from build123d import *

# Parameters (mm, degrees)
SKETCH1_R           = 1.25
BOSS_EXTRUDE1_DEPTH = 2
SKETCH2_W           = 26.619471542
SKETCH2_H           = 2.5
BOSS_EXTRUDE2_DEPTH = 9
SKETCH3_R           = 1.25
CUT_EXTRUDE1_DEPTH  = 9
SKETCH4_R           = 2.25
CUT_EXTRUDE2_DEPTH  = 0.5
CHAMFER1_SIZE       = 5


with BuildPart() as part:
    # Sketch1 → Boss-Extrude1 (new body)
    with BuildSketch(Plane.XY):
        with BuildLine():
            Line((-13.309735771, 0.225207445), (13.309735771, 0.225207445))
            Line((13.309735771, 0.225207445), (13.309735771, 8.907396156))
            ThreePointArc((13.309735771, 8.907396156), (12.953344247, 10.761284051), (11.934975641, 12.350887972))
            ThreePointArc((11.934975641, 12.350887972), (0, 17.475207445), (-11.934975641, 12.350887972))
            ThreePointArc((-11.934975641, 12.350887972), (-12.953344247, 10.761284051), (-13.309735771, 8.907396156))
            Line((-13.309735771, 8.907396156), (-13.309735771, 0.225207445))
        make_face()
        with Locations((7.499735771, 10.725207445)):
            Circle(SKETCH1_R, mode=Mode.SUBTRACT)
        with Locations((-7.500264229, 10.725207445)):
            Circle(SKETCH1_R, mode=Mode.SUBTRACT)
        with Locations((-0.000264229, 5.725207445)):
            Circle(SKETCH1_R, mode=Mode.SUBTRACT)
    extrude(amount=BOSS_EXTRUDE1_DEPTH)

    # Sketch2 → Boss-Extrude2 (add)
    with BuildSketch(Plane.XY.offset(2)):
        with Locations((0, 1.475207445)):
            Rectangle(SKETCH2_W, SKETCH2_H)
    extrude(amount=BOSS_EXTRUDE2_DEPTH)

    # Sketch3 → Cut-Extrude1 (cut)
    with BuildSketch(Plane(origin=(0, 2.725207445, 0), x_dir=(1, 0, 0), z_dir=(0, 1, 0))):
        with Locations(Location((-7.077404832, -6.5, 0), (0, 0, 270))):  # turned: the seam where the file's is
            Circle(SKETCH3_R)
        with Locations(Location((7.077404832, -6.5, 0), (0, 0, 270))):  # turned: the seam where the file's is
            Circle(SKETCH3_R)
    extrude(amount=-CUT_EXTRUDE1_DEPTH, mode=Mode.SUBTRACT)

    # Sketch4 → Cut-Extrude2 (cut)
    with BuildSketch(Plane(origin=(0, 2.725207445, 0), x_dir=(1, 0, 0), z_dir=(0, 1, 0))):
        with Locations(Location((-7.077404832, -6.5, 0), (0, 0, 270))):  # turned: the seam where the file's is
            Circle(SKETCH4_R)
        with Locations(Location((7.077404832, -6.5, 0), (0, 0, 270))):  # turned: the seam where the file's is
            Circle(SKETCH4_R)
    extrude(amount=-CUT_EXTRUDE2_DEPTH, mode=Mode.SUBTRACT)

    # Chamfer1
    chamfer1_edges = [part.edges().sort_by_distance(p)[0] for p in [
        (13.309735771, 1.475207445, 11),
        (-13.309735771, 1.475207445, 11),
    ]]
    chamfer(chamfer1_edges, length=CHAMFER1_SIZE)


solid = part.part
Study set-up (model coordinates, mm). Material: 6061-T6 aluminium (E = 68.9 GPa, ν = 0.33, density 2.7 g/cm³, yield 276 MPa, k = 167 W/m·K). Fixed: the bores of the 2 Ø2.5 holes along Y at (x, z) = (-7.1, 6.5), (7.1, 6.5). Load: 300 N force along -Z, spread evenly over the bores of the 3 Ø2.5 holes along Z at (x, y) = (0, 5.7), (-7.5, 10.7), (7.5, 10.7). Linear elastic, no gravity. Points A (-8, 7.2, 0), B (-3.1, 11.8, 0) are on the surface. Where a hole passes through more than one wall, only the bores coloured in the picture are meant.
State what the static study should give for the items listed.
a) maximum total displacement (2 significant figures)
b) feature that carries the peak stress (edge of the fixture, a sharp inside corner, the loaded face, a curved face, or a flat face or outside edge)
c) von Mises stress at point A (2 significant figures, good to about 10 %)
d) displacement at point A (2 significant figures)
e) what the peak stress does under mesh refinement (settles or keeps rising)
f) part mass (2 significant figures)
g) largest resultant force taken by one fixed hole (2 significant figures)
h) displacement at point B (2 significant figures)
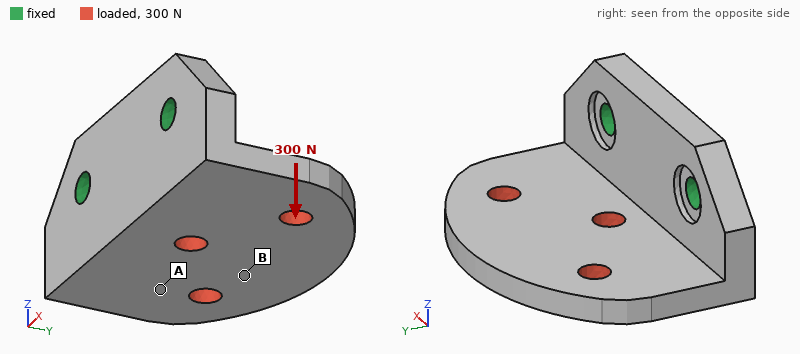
0.19 mm
edge of the fixture
43 MPa
0.063 mm
keeps rising
3.5 g
150 N
0.12 mm
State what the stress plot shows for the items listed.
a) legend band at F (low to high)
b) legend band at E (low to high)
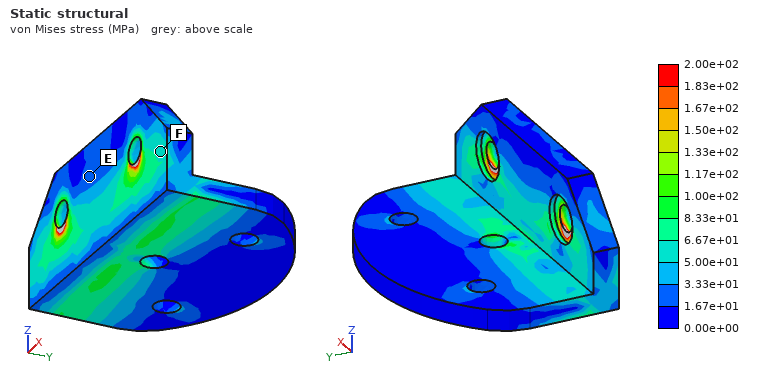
5.00e+01 to 6.67e+01 MPa
1.67e+01 to 3.33e+01 MPa
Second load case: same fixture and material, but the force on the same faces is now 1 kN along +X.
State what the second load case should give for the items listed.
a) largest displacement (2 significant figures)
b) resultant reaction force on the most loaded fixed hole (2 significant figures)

76 µm
770 N
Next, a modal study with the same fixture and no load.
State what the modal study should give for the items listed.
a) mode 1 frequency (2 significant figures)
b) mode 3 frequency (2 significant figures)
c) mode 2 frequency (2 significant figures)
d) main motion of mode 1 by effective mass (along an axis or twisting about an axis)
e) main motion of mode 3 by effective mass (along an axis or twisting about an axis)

5800 Hz
18 kHz
12 kHz
along Z
along X
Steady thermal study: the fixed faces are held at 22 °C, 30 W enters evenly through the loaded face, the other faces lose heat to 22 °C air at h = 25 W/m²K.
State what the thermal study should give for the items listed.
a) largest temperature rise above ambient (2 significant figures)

47 K
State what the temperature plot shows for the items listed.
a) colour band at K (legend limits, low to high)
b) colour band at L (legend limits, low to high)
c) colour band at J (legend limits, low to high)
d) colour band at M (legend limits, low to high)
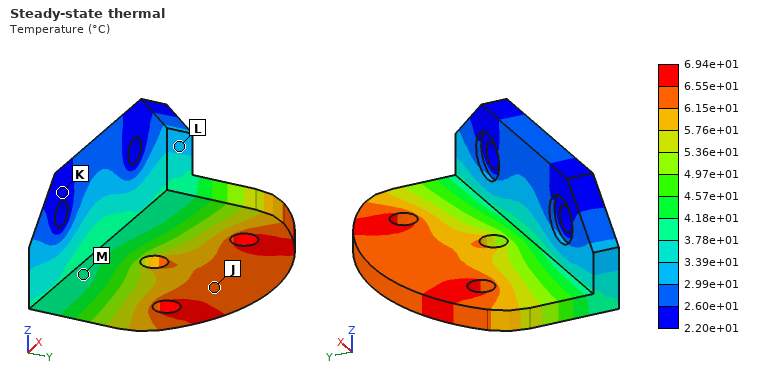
2.20e+01 to 2.60e+01 °C
2.99e+01 to 3.39e+01 °C
6.15e+01 to 6.55e+01 °C
3.78e+01 to 4.18e+01 °C
